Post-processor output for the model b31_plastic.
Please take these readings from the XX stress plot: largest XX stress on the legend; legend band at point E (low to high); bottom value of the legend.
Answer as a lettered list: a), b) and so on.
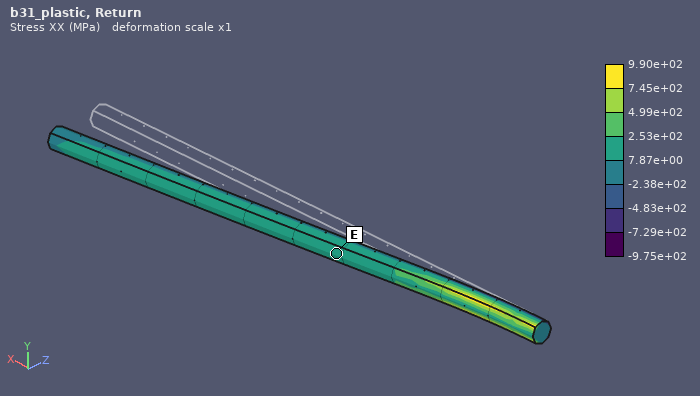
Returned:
a) 9.90e+02 MPa
b) 7.87e+00 to 2.53e+02 MPa
c) -9.75e+02 MPa
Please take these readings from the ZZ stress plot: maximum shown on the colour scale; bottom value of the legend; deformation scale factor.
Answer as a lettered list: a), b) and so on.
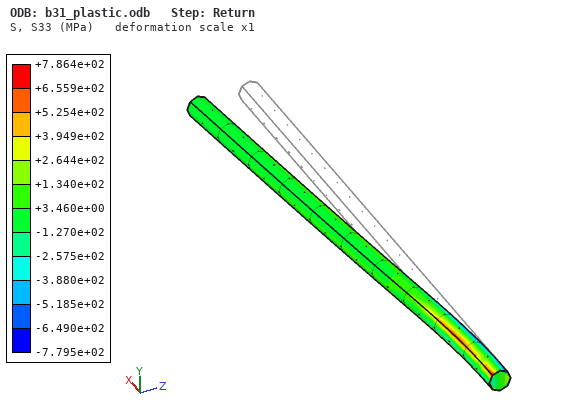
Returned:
a) +7.864e+02 MPa
b) -7.795e+02 MPa
c) 1
